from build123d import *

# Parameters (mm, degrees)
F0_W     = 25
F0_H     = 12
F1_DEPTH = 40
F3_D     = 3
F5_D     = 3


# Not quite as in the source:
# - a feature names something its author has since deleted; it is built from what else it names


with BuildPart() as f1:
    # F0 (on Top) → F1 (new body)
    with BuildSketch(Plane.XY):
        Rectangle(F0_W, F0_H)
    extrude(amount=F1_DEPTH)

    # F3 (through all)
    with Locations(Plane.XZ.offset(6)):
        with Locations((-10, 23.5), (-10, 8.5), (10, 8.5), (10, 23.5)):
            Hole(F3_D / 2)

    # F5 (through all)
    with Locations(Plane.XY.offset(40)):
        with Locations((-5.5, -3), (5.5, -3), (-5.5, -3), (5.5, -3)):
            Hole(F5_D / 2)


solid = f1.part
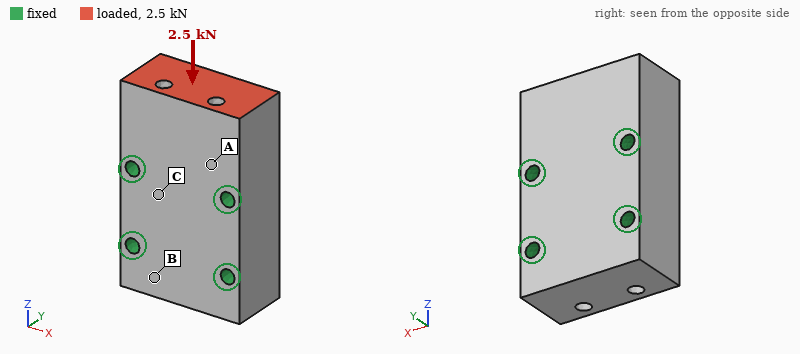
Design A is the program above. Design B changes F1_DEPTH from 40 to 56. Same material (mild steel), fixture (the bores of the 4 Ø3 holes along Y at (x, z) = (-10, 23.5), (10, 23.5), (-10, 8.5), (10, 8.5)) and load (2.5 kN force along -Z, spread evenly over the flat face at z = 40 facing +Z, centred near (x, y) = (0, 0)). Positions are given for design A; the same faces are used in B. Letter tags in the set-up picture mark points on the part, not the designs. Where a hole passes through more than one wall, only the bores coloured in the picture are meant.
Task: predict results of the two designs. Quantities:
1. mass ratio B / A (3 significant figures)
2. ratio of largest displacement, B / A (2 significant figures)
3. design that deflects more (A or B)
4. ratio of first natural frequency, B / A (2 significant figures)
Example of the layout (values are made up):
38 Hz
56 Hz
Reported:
1.41
1.8
B
0.33
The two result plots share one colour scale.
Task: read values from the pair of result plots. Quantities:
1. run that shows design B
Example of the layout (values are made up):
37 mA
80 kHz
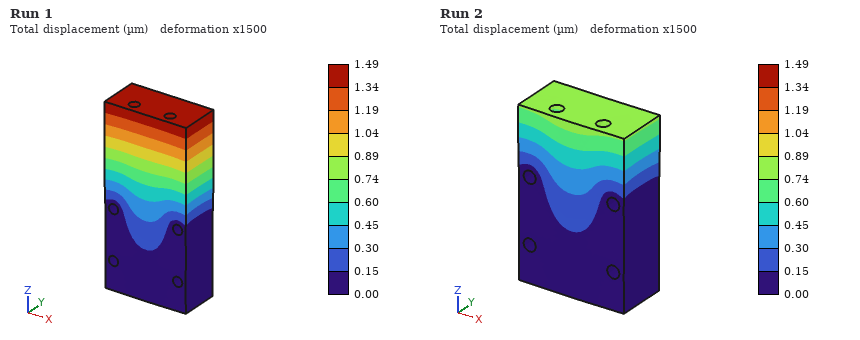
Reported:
Run 1
